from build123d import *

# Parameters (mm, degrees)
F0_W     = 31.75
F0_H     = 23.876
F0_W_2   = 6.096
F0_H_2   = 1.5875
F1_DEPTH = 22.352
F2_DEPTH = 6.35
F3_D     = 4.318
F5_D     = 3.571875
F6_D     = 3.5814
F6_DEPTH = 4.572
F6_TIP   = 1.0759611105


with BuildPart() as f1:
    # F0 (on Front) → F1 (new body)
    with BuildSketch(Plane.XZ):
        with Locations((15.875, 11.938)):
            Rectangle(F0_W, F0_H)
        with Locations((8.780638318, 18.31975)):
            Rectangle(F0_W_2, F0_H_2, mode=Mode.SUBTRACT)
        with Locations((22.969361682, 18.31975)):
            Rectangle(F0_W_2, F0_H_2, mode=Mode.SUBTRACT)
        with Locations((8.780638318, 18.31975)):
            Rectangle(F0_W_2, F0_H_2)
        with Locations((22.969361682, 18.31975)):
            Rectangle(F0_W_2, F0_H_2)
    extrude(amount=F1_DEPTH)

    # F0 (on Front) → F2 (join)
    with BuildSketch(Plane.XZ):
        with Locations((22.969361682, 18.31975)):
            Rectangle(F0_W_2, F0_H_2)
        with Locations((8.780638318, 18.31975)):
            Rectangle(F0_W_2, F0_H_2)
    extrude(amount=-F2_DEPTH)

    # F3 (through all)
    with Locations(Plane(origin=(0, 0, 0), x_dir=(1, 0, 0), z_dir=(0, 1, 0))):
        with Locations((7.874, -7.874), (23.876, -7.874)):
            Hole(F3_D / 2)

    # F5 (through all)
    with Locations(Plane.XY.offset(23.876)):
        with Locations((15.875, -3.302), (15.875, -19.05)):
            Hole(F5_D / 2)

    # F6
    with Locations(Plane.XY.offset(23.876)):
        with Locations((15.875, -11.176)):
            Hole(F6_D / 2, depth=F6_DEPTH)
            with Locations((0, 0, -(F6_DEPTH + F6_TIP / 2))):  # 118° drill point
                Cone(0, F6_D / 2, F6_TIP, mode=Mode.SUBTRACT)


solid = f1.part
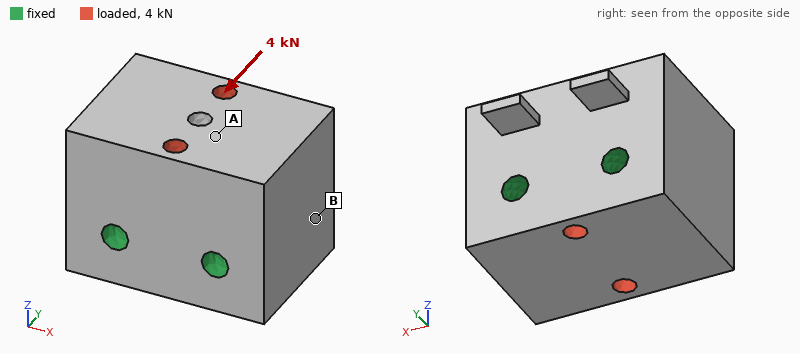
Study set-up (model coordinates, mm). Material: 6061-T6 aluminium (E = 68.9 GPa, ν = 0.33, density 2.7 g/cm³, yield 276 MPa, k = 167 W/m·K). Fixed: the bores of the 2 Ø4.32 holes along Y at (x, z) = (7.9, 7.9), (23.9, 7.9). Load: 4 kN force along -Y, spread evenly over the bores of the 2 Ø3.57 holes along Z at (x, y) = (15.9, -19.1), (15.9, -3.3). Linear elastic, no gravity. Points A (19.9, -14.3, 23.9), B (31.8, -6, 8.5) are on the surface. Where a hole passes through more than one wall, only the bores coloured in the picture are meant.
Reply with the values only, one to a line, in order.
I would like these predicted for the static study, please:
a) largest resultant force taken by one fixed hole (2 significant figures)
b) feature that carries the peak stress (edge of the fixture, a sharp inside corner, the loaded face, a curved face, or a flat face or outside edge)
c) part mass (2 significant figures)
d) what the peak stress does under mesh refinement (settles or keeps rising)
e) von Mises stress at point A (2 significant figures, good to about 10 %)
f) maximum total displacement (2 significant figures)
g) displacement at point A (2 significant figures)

2.0 kN
edge of the fixture
43 g
keeps rising
6.2 MPa
4.2 µm
2.8 µm
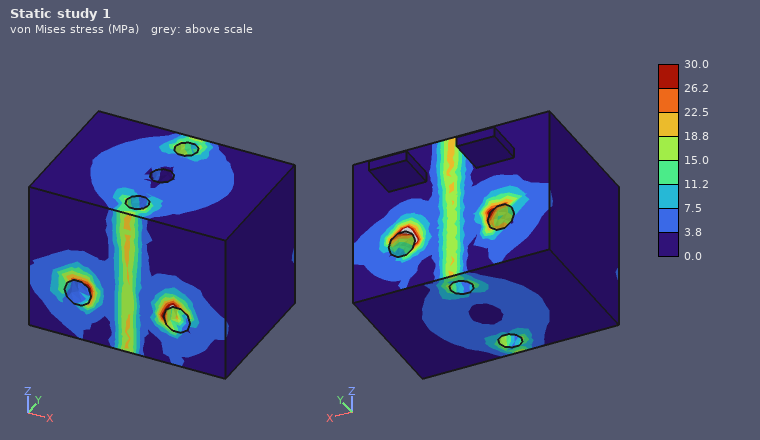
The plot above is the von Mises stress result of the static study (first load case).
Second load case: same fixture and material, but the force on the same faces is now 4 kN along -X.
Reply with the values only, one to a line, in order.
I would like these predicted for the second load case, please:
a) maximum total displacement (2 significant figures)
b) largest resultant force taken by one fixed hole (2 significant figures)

2.5 µm
2.1 kN
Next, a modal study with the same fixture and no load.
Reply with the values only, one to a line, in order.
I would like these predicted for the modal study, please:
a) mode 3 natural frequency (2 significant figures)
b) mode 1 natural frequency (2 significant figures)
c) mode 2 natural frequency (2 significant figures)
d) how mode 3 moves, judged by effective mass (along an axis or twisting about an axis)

35 kHz
28 kHz
28 kHz
along X
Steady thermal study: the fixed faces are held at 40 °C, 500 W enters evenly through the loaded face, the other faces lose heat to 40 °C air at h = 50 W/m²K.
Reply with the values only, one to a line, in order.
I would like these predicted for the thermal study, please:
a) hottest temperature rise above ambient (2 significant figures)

49 K
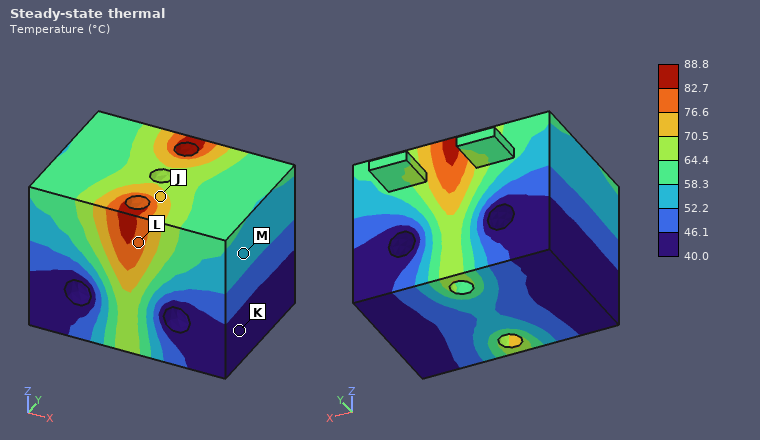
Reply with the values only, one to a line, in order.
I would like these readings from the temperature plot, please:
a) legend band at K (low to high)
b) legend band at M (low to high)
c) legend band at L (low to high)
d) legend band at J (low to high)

40.0 to 46.1 °C
52.2 to 58.3 °C
76.6 to 82.7 °C
70.5 to 76.6 °C
